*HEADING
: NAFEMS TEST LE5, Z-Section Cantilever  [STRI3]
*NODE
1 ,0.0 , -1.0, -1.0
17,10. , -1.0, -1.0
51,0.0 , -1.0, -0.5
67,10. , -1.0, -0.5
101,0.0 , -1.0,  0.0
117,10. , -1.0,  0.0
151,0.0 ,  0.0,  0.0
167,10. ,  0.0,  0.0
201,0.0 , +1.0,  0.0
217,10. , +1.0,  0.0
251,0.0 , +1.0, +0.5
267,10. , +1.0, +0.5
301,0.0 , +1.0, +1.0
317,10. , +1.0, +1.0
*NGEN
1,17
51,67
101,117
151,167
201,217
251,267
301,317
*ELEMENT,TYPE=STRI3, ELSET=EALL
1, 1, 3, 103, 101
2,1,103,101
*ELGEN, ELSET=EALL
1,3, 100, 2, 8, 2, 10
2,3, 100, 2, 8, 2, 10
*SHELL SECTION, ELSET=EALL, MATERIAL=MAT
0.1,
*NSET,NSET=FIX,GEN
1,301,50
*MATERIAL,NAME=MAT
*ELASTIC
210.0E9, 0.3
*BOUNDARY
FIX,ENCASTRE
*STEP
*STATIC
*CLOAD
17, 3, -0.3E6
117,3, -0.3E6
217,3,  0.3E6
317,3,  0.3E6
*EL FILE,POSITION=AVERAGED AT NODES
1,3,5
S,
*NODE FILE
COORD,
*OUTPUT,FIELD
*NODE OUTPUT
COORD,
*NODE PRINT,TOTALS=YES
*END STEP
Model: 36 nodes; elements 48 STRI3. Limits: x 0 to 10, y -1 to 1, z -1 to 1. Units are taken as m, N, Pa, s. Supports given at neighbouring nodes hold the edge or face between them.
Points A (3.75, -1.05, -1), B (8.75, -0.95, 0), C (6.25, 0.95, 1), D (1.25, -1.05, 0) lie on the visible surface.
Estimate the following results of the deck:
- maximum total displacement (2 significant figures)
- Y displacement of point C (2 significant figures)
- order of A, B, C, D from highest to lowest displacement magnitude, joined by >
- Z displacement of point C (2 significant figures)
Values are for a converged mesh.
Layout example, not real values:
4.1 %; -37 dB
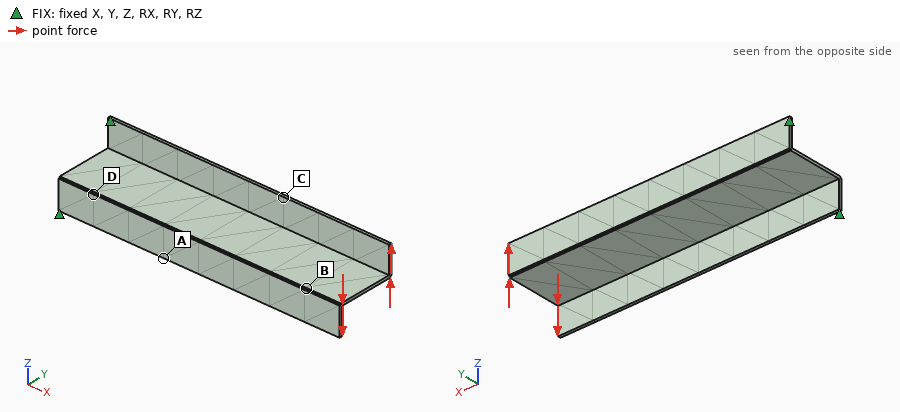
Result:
0.17 m; -0.076 m; C > B > A > D; 0.072 m
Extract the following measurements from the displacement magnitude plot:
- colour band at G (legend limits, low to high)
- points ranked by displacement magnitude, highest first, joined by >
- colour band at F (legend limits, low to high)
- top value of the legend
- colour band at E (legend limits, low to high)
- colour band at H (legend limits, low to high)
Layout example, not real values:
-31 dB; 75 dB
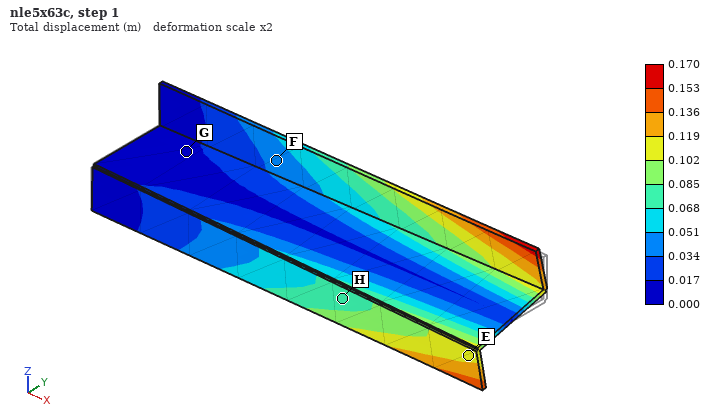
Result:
0.000 to 0.017 m; E > H > F > G; 0.034 to 0.051 m; 0.170 m; 0.102 to 0.119 m; 0.068 to 0.085 m
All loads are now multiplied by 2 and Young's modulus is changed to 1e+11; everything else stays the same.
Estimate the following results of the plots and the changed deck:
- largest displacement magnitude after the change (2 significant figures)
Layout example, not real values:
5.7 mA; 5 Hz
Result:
0.71 m
